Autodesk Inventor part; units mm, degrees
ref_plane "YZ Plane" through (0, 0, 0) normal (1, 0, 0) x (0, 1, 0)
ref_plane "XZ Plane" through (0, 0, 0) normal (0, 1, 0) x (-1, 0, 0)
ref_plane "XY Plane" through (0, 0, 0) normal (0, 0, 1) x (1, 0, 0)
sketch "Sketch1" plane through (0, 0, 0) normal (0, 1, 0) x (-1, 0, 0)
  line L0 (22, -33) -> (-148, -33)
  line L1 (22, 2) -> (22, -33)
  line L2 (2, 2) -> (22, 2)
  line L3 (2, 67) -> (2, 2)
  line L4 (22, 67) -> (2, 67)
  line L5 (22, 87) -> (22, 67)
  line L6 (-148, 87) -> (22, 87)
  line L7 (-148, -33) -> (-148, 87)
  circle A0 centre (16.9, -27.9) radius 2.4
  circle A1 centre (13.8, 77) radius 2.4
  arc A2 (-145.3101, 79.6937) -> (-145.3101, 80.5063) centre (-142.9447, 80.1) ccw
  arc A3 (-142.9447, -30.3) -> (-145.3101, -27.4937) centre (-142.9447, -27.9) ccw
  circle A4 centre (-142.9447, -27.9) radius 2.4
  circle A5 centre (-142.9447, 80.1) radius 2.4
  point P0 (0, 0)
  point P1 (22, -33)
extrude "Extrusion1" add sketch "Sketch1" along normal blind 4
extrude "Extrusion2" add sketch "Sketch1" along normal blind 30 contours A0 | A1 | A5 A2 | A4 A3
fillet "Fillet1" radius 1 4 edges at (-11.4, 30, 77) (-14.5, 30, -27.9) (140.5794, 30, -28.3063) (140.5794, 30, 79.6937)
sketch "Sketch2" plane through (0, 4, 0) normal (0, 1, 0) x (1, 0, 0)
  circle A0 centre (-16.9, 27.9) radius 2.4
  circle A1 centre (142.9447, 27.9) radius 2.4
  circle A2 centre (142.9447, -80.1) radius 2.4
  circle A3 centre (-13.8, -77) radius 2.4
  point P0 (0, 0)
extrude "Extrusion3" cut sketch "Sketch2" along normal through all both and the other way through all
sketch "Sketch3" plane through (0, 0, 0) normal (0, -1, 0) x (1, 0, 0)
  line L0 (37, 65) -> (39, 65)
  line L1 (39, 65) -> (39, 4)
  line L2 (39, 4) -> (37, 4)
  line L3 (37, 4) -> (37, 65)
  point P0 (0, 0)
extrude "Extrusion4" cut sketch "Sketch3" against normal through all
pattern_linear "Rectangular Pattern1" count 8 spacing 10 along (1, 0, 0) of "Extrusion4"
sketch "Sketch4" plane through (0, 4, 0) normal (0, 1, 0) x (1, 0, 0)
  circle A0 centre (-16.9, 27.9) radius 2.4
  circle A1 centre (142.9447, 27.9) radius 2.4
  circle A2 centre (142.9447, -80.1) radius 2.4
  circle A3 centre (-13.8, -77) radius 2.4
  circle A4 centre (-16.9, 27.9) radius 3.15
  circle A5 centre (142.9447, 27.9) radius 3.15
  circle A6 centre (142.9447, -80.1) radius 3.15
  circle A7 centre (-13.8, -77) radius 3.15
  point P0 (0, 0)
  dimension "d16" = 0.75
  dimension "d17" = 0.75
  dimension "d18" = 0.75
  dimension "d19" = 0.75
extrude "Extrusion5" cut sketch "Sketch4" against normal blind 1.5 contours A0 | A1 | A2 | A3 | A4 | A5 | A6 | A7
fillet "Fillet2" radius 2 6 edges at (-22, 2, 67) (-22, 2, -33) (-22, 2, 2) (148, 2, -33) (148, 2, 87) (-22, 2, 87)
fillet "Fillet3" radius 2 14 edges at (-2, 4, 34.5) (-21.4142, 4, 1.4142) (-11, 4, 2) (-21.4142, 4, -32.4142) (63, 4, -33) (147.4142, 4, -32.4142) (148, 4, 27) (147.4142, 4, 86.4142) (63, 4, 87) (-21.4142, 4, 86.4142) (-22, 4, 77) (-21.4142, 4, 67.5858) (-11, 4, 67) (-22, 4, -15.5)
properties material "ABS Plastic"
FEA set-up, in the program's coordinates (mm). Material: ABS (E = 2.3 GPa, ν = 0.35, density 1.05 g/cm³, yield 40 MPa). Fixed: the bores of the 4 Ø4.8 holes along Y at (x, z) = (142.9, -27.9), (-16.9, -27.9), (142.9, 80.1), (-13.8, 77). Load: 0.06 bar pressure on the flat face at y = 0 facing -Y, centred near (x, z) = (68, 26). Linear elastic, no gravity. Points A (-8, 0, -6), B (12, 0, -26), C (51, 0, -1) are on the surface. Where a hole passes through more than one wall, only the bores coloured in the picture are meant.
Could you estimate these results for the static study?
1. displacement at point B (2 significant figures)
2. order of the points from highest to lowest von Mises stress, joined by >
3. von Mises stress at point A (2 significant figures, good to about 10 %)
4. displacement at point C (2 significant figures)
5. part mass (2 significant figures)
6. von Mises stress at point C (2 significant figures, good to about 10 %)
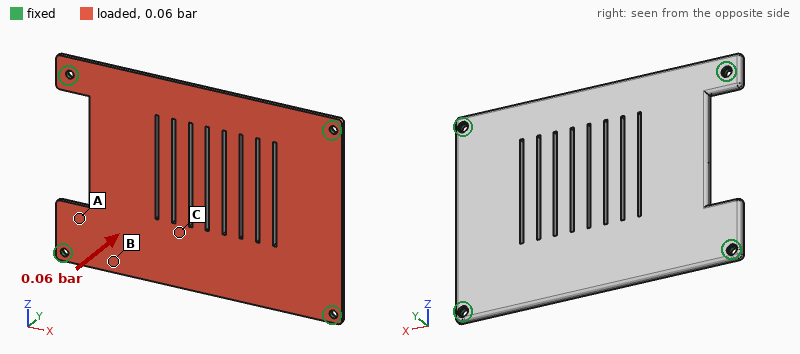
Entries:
0.79 mm
C > A > B
2.1 MPa
2.1 mm
75 g
4.0 MPa
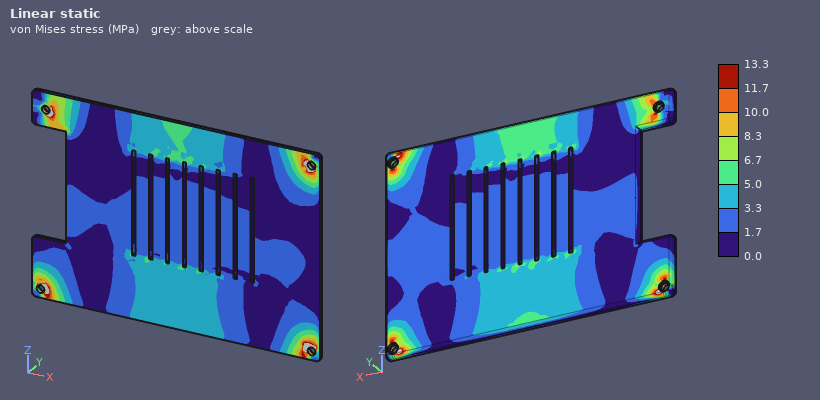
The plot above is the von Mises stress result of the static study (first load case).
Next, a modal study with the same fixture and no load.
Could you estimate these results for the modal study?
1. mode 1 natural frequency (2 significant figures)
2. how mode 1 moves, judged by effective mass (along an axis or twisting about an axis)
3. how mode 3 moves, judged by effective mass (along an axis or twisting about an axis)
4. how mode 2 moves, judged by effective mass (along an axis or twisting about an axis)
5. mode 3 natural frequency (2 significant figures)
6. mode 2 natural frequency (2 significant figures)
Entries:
150 Hz
along Y
twisting about Z
twisting about X
350 Hz
280 Hz
